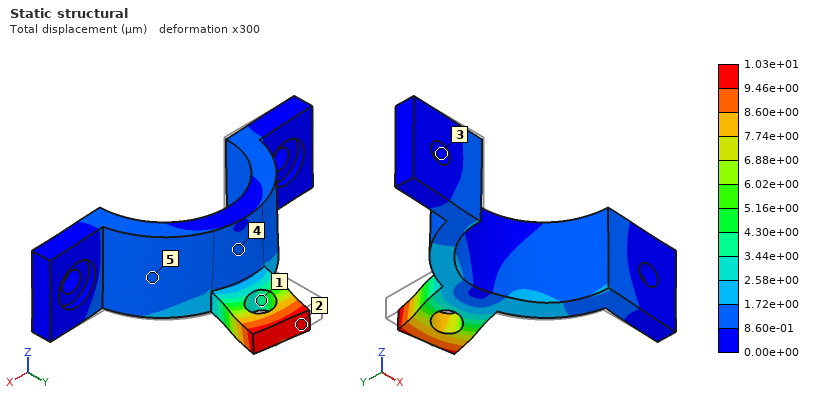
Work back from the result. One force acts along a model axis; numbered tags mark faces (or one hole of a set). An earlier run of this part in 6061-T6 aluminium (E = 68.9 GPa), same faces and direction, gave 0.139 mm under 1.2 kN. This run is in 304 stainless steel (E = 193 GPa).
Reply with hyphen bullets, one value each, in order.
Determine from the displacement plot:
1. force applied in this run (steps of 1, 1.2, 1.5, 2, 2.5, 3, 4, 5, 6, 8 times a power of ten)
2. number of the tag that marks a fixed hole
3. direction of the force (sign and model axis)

- 250 N
- 3
- +X
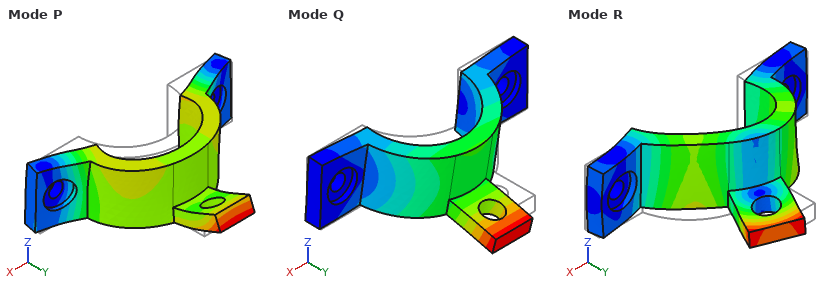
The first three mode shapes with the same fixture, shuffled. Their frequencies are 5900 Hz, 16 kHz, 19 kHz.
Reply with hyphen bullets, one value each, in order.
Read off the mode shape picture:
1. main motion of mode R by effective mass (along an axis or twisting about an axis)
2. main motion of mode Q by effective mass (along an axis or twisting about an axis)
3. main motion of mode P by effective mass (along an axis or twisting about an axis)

- along X
- along Z
- along Y
